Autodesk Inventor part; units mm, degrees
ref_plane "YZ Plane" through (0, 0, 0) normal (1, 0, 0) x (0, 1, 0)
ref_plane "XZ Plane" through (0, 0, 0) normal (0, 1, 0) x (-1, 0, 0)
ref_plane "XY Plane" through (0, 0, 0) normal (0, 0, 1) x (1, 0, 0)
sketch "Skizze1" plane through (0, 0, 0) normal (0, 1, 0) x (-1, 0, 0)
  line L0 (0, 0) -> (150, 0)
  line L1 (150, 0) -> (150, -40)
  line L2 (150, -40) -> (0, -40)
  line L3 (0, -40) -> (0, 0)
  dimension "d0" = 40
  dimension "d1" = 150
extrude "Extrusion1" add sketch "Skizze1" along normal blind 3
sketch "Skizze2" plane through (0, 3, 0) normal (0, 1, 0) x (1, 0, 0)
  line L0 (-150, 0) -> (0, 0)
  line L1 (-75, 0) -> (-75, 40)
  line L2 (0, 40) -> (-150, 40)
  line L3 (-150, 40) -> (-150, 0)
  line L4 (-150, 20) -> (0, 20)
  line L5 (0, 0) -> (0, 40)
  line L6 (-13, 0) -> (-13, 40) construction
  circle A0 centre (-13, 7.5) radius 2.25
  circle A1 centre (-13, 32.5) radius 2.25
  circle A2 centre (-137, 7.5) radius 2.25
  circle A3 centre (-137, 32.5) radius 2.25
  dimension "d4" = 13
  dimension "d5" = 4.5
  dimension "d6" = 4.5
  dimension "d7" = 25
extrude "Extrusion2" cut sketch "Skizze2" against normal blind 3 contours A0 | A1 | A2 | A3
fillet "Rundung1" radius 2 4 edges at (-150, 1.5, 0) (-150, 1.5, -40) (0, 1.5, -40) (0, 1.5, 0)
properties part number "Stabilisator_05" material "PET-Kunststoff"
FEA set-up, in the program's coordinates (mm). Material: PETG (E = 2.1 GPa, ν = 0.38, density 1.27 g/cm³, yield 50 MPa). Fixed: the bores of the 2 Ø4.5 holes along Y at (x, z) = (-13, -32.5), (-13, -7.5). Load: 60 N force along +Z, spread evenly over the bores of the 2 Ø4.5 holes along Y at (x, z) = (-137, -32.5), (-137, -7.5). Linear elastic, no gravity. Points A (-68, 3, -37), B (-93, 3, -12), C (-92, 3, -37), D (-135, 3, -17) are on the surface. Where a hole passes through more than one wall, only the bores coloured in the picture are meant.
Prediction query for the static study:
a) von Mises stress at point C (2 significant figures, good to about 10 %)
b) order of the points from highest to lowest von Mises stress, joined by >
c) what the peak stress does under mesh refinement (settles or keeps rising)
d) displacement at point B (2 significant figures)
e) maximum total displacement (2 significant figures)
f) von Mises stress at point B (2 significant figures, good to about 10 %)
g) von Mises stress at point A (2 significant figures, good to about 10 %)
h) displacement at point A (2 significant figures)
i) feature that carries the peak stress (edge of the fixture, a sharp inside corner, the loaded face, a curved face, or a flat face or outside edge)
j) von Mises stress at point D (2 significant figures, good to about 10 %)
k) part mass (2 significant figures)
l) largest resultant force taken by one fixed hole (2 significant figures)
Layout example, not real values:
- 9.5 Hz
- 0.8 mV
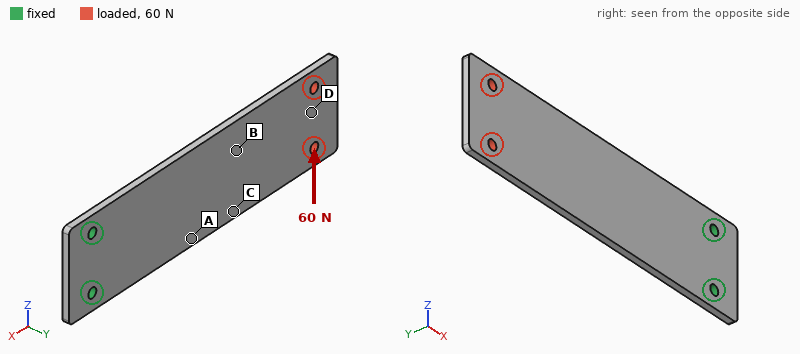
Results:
- 2.9 MPa
- A > C > B > D
- keeps rising
- 0.67 mm
- 1.5 mm
- 1.7 MPa
- 4.3 MPa
- 0.40 mm
- edge of the fixture
- 0.88 MPa
- 23 g
- 280 N
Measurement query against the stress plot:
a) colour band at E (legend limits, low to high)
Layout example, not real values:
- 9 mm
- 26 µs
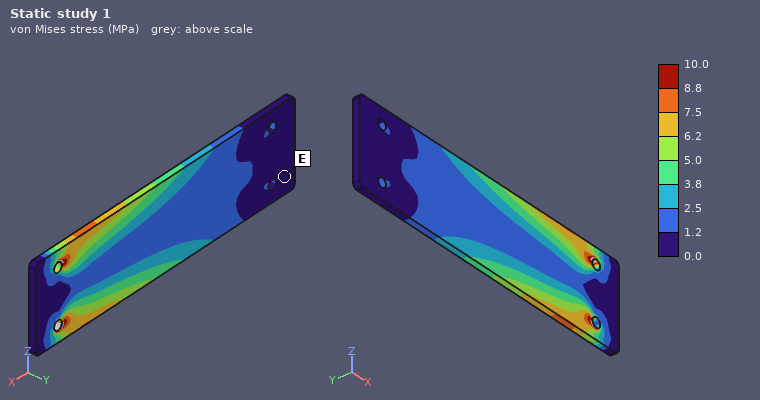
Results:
- 0.0 to 1.2 MPa
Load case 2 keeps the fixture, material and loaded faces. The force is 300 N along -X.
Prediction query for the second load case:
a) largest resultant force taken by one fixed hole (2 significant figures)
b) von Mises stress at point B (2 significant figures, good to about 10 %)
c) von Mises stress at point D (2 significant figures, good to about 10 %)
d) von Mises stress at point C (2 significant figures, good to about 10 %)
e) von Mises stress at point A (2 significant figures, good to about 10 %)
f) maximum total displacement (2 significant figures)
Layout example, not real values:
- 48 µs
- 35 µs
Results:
- 150 N
- 2.5 MPa
- 1.4 MPa
- 2.5 MPa
- 2.5 MPa
- 0.16 mm
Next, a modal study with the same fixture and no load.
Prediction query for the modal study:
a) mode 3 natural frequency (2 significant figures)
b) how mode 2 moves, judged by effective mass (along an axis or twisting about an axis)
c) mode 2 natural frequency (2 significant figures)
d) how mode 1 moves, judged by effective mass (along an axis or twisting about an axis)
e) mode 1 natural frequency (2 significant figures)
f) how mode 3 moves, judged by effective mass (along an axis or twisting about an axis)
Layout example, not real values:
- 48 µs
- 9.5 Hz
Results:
- 230 Hz
- along Y
- 210 Hz
- along Y
- 34 Hz
- twisting about X
